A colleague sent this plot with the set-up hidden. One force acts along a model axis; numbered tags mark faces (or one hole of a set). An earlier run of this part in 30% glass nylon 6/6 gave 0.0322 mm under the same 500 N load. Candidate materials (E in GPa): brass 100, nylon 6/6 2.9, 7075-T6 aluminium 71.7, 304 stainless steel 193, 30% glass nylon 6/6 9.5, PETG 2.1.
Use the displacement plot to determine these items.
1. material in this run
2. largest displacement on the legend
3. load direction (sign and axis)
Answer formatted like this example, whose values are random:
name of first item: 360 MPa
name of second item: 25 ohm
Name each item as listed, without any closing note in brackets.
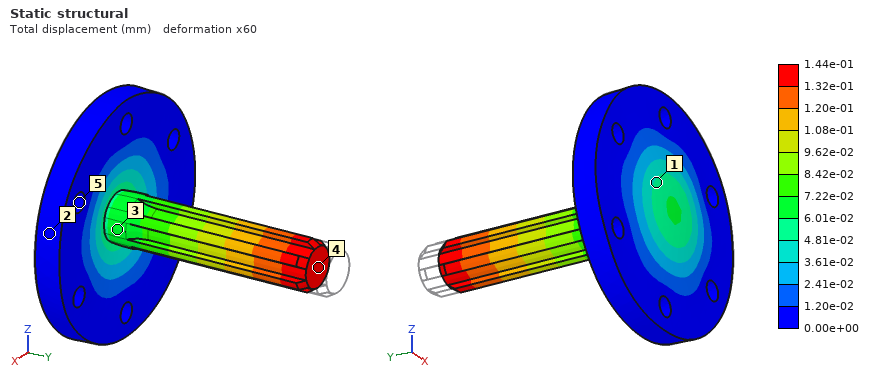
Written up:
material in this run: PETG
largest displacement on the legend: 1.44e-01 mm
load direction: -Y
